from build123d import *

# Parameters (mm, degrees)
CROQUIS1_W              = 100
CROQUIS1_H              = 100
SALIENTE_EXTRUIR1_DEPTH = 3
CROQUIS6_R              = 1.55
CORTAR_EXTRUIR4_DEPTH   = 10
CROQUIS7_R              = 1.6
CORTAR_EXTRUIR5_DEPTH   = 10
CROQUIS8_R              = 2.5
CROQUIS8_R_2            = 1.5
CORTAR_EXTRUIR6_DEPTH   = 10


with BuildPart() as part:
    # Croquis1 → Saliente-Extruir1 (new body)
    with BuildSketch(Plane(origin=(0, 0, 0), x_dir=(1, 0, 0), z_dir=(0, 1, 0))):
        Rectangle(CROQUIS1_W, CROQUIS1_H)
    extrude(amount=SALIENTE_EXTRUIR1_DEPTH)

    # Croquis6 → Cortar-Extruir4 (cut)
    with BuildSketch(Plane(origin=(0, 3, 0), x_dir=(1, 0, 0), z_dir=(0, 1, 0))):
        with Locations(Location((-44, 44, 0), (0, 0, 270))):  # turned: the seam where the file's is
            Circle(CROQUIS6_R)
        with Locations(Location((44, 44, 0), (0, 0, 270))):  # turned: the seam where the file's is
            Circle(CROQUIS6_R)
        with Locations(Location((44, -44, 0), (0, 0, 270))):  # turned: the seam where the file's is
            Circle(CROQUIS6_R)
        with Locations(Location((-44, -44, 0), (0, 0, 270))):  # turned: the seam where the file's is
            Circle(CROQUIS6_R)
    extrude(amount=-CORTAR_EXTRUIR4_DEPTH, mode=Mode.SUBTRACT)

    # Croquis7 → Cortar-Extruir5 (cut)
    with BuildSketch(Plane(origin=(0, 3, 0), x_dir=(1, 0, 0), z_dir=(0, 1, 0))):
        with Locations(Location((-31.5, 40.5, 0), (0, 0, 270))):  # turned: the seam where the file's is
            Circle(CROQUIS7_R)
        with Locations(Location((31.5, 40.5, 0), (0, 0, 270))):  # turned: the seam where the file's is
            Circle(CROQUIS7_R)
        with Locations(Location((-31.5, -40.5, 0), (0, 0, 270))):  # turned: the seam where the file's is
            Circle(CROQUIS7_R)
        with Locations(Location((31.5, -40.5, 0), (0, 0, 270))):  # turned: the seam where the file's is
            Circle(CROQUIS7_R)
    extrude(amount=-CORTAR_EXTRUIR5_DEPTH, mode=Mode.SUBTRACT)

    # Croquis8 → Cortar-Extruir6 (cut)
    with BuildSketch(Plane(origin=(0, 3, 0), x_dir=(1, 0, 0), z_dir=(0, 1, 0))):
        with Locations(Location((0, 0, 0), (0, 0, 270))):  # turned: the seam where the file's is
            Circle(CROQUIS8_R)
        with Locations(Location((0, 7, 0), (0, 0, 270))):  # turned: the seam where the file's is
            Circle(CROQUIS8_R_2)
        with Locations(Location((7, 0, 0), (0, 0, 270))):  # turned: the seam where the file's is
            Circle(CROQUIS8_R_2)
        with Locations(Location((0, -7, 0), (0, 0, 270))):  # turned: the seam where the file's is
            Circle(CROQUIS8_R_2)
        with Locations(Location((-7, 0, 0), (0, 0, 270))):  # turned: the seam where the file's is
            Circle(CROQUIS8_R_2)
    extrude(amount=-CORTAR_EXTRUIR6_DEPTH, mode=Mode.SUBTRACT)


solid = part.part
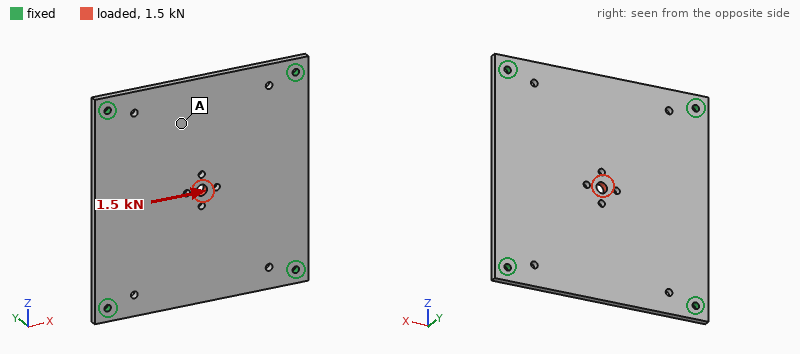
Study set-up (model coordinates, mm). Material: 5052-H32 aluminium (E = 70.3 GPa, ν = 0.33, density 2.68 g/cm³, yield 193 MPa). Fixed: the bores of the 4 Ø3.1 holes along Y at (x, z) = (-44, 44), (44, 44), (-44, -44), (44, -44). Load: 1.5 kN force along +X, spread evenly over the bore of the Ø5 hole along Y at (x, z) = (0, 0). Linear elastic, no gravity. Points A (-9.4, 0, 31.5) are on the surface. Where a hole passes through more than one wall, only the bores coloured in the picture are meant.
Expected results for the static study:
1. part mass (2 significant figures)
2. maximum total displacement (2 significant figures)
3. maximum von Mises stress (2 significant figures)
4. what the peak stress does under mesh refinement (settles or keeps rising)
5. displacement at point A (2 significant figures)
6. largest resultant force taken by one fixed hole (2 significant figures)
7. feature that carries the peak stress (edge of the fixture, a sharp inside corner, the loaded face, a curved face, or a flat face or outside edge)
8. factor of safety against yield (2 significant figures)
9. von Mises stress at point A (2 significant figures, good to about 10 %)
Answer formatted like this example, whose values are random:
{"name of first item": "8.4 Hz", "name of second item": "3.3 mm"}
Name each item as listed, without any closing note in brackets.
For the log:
{"part mass": "80 g", "maximum total displacement": "11 µm", "maximum von Mises stress": "57 MPa", "what the peak stress does under mesh refinement": "settles", "displacement at point A": "3.4 µm", "largest resultant force taken by one fixed hole": "430 N", "feature that carries the peak stress": "the loaded face", "factor of safety against yield": "3.4", "von Mises stress at point A": "3.8 MPa"}
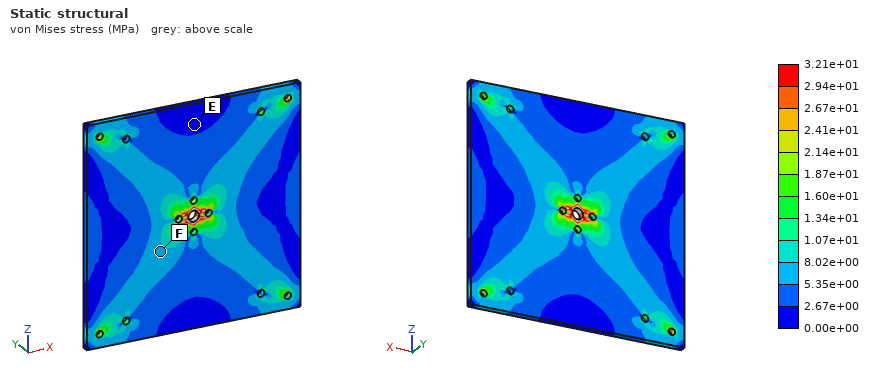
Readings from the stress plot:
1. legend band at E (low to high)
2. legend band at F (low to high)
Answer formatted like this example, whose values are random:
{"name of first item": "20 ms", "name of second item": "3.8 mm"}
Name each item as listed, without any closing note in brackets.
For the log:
{"legend band at E": "0.00e+00 to 2.67e+00 MPa", "legend band at F": "5.35e+00 to 8.02e+00 MPa"}
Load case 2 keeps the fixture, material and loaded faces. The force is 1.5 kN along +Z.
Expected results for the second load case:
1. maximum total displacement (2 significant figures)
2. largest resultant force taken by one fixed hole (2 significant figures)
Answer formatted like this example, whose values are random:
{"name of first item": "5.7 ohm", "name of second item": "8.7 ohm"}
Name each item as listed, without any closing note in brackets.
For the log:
{"maximum total displacement": "11 µm", "largest resultant force taken by one fixed hole": "420 N"}
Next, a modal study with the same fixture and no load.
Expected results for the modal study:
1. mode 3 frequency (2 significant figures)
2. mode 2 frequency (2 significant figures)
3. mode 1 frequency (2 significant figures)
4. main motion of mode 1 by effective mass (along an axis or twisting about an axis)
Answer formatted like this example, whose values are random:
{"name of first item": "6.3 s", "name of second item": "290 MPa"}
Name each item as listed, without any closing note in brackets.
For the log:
{"mode 3 frequency": "2200 Hz", "mode 2 frequency": "2200 Hz", "mode 1 frequency": "1200 Hz", "main motion of mode 1 by effective mass": "along Y"}
